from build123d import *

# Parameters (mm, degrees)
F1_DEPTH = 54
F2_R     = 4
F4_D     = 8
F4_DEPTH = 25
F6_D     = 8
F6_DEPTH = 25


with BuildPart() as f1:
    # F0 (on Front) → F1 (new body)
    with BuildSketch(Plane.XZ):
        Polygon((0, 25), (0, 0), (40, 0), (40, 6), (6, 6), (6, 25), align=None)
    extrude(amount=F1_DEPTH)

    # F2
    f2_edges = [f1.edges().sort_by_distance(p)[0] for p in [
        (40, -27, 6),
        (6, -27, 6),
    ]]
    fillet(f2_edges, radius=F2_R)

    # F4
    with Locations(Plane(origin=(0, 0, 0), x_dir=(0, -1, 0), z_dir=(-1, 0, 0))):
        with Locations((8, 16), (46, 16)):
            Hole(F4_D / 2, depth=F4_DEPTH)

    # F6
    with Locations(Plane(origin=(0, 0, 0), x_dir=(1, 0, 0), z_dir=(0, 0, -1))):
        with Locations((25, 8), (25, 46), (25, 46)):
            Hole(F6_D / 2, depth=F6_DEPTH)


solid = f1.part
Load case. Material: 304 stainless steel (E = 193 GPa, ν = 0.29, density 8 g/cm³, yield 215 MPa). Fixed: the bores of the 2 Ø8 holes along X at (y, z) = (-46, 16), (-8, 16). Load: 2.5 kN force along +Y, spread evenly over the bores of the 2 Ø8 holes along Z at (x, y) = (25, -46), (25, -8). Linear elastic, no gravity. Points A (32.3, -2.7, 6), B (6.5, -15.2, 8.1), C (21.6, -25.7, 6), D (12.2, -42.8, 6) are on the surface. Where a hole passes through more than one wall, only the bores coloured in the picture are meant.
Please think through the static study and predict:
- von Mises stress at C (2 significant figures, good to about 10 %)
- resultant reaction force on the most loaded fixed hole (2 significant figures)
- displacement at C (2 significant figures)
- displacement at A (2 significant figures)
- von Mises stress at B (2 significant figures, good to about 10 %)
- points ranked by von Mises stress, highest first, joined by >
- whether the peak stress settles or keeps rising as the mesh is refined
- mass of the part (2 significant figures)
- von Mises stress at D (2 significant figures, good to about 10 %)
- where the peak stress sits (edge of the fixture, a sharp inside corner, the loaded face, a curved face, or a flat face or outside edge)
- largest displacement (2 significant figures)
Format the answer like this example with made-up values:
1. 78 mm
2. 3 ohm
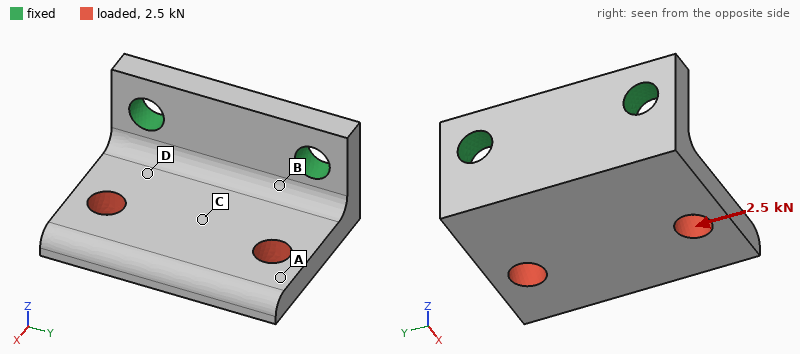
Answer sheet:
1. 20 MPa
2. 2.0 kN
3. 9.0 µm
4. 18 µm
5. 56 MPa
6. B > D > C > A
7. keeps rising
8. 140 g
9. 36 MPa
10. edge of the fixture
11. 20 µm
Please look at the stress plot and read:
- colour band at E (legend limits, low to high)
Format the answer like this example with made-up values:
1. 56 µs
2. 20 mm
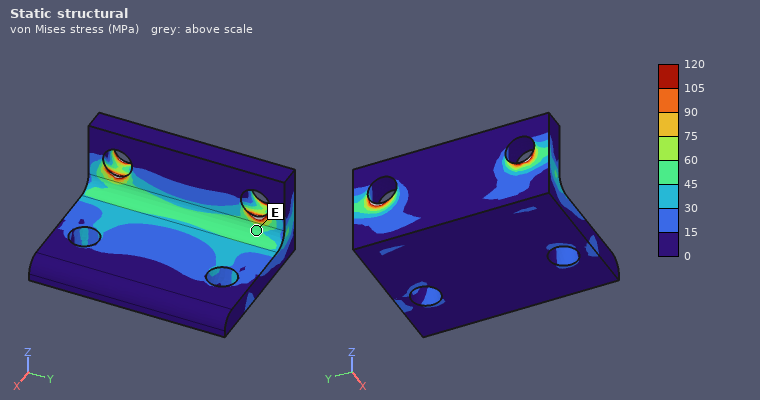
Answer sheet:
1. 45 to 60 MPa
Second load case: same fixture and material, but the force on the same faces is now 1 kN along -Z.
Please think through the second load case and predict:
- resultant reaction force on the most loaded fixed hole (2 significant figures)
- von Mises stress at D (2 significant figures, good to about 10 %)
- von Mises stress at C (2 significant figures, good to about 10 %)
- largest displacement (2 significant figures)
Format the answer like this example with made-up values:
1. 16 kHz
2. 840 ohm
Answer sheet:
1. 510 N
2. 36 MPa
3. 15 MPa
4. 68 µm
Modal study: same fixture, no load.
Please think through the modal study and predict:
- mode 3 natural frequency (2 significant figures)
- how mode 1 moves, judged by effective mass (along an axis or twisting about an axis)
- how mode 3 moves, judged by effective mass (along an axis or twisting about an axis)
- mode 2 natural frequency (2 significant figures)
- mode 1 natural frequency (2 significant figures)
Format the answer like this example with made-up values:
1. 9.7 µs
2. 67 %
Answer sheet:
1. 8900 Hz
2. along Z
3. along Y
4. 5600 Hz
5. 2700 Hz
